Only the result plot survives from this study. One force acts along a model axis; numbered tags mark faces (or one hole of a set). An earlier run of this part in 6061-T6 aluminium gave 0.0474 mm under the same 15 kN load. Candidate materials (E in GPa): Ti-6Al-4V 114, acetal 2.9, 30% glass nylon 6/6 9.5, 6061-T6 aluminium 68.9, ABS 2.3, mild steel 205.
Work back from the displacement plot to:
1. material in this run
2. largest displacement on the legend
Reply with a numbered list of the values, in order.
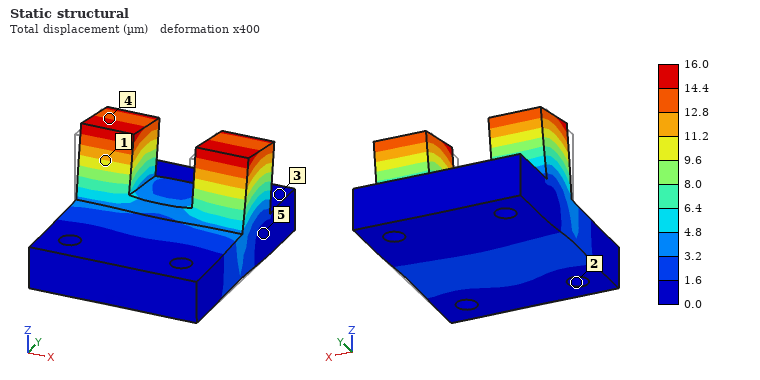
1. mild steel
2. 16.0 µm
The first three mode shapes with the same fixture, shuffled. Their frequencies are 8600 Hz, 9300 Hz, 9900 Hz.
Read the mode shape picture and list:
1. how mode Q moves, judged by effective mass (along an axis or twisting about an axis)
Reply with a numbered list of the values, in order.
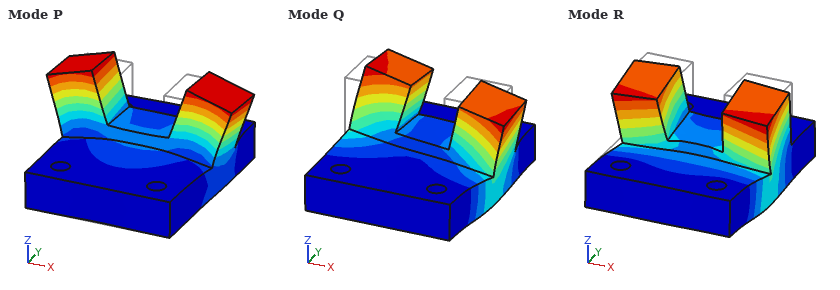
1. along X
